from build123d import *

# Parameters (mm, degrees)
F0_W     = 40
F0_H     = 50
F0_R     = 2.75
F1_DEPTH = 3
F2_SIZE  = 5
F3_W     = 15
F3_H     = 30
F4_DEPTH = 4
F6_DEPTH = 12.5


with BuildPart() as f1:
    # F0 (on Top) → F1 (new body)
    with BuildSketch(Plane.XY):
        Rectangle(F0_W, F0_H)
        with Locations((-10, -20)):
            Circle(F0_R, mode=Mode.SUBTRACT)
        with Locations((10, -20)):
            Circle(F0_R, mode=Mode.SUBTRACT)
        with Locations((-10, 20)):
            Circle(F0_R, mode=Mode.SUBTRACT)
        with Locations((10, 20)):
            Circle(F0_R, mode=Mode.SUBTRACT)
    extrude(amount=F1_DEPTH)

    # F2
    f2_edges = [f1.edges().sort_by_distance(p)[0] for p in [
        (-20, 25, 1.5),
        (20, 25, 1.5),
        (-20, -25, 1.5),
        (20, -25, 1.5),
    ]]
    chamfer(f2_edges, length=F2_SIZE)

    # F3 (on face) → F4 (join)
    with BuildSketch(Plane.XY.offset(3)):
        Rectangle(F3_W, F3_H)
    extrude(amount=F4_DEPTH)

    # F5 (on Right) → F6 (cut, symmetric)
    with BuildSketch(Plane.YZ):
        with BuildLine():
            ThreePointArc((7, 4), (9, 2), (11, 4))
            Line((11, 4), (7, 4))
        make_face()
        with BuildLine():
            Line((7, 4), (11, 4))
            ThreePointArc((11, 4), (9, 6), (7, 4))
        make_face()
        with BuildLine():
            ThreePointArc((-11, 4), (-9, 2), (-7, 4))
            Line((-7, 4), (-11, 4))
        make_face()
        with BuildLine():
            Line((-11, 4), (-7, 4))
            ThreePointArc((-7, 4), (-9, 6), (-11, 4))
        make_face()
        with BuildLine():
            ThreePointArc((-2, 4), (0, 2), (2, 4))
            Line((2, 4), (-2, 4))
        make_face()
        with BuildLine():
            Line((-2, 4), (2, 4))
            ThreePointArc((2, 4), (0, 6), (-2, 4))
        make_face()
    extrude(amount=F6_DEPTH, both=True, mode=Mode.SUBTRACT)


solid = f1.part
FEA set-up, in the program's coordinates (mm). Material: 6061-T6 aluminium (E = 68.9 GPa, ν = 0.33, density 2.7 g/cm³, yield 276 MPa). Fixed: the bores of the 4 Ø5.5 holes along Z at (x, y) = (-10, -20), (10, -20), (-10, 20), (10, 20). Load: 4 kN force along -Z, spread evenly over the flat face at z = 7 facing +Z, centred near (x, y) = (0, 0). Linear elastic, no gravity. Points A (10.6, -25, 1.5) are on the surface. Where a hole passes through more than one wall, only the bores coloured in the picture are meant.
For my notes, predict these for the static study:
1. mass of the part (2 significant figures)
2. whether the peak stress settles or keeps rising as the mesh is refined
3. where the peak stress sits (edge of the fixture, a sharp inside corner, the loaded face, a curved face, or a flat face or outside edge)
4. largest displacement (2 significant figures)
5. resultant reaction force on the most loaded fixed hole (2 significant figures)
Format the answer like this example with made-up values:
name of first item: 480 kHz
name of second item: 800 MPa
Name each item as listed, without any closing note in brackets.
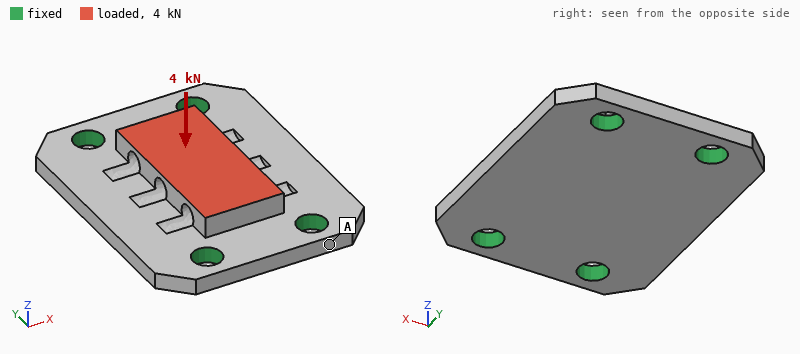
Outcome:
mass of the part: 18 g
whether the peak stress settles or keeps rising as the mesh is refined: keeps rising
where the peak stress sits: edge of the fixture
largest displacement: 64 µm
resultant reaction force on the most loaded fixed hole: 1.1 kN
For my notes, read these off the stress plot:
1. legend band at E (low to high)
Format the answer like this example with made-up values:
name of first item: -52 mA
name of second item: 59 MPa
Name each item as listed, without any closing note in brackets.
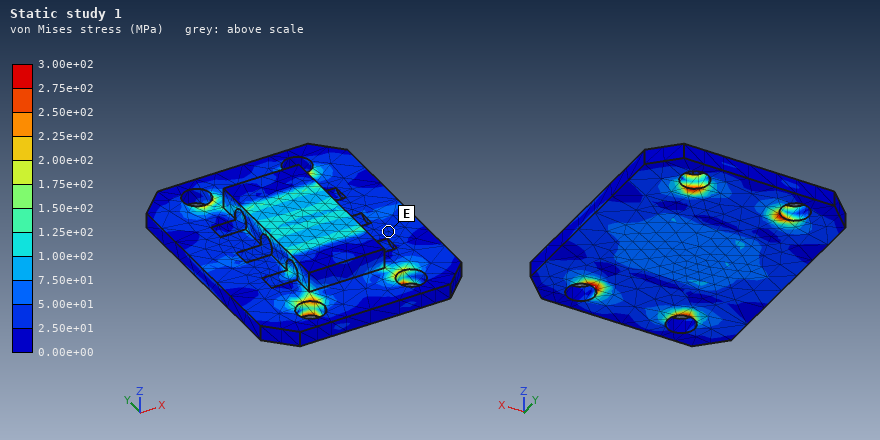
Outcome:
legend band at E: 2.50e+01 to 5.00e+01 MPa
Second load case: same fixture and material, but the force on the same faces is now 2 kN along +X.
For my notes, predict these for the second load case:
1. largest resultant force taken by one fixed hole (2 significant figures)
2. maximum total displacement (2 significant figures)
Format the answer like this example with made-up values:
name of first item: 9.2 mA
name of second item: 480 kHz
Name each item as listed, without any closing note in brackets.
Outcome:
largest resultant force taken by one fixed hole: 640 N
maximum total displacement: 17 µm
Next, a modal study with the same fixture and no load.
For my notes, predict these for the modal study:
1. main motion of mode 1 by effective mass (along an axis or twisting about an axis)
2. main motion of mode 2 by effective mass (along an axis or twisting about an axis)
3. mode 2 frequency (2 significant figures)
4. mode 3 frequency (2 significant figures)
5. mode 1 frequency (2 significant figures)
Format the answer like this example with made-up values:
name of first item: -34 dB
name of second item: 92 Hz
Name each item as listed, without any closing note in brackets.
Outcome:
main motion of mode 1 by effective mass: along Z
main motion of mode 2 by effective mass: twisting about Y
mode 2 frequency: 13 kHz
mode 3 frequency: 19 kHz
mode 1 frequency: 12 kHz
